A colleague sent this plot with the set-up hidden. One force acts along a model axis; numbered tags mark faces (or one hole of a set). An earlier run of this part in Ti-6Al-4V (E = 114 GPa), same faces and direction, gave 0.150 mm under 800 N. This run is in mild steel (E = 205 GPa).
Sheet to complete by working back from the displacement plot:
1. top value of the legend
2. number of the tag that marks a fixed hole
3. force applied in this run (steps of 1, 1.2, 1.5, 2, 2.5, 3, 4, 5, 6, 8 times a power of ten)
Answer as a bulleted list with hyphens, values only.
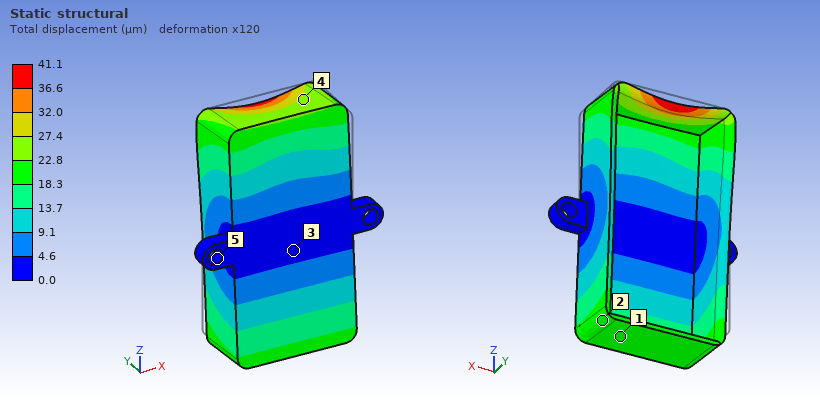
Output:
- 41.1 µm
- 5
- 400 N
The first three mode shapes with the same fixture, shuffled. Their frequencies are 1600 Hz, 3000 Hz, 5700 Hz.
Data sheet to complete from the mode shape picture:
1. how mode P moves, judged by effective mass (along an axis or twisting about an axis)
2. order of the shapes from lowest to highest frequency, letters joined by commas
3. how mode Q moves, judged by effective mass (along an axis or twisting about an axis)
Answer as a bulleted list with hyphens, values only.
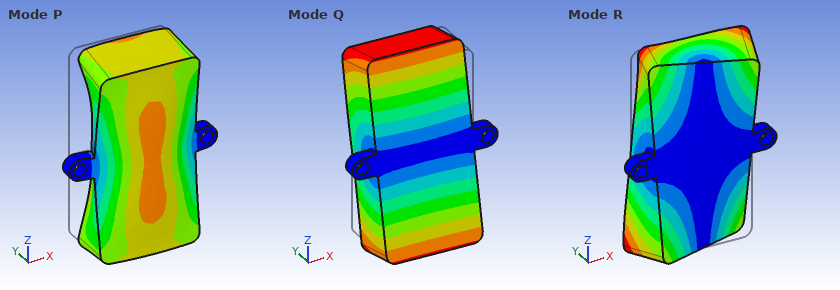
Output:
- along Y
- Q, R, P
- twisting about X
